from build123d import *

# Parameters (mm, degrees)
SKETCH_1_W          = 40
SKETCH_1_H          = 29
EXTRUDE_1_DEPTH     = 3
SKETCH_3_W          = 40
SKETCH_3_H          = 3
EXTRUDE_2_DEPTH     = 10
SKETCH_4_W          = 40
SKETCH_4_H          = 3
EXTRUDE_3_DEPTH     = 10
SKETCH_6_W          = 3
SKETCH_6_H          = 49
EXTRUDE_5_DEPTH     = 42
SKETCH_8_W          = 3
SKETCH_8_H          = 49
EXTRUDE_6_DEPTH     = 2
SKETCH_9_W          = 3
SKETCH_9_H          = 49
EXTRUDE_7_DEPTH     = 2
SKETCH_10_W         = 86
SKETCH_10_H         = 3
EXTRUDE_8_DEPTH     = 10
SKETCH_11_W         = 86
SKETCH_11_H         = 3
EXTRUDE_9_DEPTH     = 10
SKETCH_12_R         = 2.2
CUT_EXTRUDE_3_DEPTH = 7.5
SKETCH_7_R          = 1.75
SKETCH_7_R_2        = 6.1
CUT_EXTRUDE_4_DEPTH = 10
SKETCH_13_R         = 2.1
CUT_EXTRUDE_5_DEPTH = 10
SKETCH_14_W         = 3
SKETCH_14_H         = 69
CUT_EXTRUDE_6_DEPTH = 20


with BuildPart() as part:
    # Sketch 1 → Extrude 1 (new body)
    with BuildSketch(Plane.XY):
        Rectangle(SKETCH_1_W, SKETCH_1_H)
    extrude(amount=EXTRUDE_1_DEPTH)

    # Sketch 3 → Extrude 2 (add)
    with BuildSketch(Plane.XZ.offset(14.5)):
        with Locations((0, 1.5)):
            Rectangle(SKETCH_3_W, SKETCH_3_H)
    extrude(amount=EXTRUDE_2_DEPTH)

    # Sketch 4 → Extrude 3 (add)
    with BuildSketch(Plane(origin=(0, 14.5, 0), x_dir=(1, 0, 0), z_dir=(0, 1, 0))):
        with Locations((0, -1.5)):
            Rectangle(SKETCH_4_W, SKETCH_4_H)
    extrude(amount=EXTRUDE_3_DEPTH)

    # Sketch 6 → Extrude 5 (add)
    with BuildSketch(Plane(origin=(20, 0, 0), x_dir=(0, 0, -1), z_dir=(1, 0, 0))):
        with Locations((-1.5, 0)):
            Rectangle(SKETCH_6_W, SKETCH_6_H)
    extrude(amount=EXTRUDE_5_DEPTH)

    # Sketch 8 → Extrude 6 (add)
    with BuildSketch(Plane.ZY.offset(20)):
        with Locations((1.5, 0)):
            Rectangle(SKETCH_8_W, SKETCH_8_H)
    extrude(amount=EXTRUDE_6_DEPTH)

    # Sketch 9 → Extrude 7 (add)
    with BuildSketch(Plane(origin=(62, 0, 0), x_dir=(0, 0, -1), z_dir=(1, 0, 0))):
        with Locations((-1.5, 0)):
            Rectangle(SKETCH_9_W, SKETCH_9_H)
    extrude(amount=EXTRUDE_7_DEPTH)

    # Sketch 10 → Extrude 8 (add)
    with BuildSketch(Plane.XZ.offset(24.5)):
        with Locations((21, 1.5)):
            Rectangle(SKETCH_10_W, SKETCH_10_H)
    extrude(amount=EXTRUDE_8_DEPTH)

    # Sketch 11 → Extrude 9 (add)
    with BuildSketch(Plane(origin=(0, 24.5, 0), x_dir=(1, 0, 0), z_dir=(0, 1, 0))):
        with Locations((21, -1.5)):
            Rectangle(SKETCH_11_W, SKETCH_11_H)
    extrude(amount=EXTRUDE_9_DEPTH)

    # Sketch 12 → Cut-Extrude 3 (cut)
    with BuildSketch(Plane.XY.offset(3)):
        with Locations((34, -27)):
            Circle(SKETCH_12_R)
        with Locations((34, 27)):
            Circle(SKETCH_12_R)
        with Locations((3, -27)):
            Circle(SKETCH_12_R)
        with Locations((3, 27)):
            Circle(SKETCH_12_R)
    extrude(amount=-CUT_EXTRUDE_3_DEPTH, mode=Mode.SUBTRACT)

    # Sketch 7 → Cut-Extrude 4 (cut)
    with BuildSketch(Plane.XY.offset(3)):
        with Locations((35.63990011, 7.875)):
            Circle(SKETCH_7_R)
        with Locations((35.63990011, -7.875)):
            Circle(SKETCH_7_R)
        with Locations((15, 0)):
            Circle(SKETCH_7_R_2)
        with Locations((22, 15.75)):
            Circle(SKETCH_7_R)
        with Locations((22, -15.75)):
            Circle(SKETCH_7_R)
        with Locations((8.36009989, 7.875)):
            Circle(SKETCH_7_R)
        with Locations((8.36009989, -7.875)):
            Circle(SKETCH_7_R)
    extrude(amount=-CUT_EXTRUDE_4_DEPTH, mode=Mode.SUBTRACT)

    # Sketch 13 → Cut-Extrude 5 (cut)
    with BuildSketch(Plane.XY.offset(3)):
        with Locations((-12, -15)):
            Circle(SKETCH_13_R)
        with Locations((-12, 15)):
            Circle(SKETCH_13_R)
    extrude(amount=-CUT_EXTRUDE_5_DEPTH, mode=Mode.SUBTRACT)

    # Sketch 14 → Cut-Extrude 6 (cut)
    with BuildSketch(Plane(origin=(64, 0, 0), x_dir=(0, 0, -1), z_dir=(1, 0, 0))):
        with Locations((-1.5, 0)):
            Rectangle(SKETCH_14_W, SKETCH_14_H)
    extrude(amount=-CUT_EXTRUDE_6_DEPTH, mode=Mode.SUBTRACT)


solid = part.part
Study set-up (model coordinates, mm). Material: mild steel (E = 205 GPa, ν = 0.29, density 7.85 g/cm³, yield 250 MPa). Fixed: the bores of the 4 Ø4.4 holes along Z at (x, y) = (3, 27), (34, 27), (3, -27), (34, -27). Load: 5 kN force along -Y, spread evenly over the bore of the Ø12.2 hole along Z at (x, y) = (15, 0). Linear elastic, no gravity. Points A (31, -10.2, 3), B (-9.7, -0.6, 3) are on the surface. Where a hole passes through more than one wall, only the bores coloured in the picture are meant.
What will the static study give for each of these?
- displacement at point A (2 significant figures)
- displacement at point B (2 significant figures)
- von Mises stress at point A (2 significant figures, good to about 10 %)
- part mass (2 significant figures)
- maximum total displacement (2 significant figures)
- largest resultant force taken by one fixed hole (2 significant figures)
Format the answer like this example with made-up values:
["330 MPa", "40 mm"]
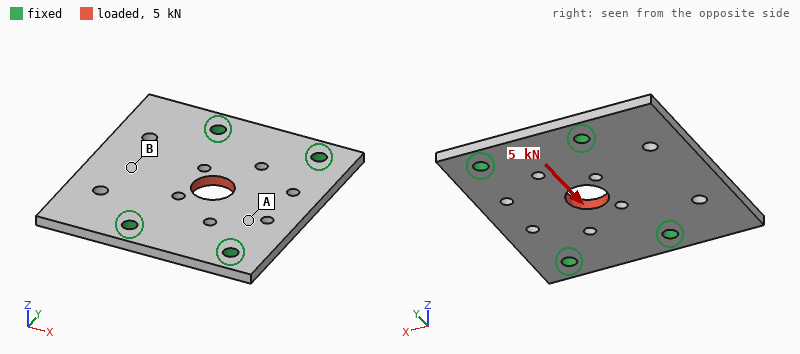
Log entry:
["1.7 µm", "1.3 µm", "15 MPa", "100 g", "4.9 µm", "1.5 kN"]
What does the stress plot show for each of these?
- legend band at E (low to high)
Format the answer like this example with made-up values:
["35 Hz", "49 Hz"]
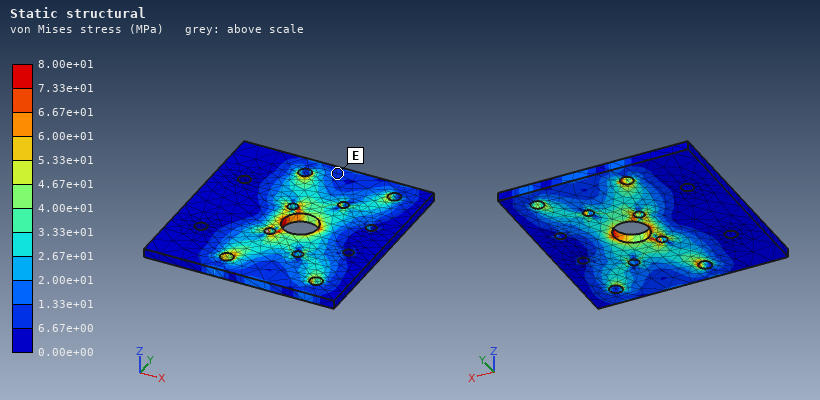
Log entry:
["6.67e+00 to 1.33e+01 MPa"]
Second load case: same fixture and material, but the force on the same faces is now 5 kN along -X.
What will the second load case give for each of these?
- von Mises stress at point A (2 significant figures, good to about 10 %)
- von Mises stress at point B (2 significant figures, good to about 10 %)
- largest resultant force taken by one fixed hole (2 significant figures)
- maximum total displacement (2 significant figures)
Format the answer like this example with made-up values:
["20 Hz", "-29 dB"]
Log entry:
["27 MPa", "16 MPa", "1.5 kN", "7.0 µm"]
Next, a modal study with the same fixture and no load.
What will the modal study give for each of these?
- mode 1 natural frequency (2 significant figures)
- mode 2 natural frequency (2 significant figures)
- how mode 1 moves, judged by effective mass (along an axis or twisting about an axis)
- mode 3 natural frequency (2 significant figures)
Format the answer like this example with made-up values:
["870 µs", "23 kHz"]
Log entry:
["3100 Hz", "5200 Hz", "along Z", "5300 Hz"]
